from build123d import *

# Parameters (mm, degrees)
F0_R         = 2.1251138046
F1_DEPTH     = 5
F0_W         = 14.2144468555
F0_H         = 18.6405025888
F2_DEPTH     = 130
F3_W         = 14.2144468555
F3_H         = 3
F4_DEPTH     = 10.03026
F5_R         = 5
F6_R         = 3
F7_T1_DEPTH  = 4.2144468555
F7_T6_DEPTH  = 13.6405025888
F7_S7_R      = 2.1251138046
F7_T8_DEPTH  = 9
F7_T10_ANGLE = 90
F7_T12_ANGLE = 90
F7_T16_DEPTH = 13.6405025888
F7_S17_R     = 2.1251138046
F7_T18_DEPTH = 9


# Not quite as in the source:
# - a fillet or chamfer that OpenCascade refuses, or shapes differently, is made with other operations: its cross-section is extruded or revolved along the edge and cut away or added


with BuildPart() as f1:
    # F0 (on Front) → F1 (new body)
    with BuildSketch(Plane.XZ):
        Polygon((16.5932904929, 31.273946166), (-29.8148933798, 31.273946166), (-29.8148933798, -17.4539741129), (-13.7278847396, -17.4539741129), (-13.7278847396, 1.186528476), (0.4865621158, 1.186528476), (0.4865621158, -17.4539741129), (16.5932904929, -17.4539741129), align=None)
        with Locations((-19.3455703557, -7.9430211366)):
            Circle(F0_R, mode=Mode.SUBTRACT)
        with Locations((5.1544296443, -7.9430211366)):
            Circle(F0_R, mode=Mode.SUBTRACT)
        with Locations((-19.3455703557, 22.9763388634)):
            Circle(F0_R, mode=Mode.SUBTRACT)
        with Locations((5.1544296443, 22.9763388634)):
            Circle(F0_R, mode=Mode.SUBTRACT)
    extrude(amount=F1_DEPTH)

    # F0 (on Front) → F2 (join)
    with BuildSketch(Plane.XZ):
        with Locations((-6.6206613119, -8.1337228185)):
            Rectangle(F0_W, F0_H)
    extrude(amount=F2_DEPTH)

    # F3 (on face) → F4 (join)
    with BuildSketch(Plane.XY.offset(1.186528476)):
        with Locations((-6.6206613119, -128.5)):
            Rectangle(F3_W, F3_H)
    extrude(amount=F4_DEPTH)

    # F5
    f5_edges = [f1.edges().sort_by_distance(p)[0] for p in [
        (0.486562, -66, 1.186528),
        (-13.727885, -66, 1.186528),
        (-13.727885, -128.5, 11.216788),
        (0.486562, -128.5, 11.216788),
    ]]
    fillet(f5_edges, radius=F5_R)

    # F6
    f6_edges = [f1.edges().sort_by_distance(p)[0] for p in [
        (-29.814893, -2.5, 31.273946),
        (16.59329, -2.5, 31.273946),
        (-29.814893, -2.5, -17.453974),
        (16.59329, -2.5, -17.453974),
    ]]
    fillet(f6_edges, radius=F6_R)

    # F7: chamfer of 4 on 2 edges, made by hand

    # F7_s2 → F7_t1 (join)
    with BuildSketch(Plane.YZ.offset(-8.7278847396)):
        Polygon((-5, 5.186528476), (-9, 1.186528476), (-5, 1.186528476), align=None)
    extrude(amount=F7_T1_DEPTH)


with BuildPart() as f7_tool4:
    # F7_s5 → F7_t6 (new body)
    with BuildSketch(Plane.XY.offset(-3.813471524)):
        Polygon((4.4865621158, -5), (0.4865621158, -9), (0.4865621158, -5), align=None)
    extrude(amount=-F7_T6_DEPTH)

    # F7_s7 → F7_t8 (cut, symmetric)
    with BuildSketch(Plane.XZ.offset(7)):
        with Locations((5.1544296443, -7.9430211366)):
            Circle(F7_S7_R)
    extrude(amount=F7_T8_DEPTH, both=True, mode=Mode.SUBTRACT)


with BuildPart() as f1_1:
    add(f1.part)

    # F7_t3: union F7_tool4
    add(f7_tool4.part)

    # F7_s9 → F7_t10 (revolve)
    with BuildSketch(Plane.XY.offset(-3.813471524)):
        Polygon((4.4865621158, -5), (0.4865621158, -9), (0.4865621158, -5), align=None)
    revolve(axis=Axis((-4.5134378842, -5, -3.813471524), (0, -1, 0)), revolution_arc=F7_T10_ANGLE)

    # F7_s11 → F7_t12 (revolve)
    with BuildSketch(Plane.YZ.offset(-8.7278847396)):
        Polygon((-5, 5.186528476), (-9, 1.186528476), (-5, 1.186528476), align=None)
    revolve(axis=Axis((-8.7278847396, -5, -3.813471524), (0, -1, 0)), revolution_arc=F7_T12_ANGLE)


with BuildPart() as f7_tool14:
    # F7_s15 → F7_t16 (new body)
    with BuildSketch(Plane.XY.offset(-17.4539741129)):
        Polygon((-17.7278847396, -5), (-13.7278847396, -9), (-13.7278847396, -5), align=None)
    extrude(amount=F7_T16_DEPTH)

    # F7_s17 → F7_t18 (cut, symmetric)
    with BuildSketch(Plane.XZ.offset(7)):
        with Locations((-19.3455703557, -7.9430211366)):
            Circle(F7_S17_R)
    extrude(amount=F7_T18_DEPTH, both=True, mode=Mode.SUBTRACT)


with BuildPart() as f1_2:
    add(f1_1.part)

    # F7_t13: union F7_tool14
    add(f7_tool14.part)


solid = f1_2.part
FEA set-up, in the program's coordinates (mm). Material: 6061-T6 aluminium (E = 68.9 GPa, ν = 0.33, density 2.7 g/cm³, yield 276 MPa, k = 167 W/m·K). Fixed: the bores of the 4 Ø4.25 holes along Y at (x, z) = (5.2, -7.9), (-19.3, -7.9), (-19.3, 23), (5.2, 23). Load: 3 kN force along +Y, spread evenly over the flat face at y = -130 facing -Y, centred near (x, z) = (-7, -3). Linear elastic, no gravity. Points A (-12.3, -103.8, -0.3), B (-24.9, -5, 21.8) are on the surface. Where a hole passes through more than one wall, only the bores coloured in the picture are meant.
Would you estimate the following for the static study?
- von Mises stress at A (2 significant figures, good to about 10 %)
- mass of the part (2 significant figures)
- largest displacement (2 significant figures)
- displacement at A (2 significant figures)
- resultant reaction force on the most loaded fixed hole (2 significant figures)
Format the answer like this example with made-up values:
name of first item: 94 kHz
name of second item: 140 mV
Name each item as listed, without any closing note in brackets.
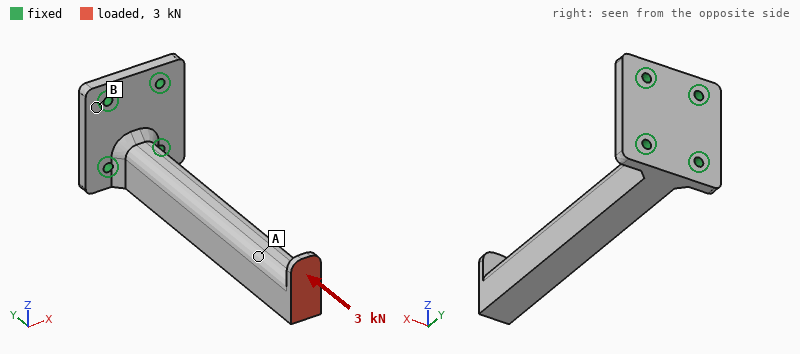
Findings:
von Mises stress at A: 30 MPa
mass of the part: 120 g
largest displacement: 0.39 mm
displacement at A: 0.21 mm
resultant reaction force on the most loaded fixed hole: 1.5 kN
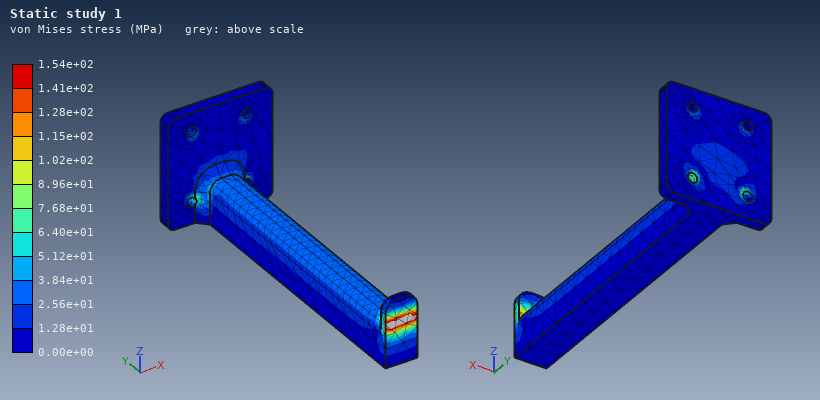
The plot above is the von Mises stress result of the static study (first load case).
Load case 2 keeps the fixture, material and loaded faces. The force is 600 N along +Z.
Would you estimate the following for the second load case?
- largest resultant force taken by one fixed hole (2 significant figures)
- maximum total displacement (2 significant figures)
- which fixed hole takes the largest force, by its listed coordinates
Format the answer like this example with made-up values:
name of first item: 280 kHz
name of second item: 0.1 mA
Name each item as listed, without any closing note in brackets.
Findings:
largest resultant force taken by one fixed hole: 1.1 kN
maximum total displacement: 1.3 mm
which fixed hole takes the largest force, by its listed coordinates: (5.2, -7.9)
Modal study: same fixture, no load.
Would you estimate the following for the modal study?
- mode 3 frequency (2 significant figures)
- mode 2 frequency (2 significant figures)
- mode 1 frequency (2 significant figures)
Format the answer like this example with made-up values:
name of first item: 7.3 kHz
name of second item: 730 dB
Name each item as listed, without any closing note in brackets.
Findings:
mode 3 frequency: 4000 Hz
mode 2 frequency: 680 Hz
mode 1 frequency: 670 Hz
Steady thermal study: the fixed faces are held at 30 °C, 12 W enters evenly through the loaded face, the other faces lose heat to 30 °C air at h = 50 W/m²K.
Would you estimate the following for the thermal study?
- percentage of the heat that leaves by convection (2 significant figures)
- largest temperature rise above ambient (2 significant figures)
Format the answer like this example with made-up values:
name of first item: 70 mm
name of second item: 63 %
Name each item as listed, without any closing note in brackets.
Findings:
percentage of the heat that leaves by convection: 43 %
largest temperature rise above ambient: 30 K
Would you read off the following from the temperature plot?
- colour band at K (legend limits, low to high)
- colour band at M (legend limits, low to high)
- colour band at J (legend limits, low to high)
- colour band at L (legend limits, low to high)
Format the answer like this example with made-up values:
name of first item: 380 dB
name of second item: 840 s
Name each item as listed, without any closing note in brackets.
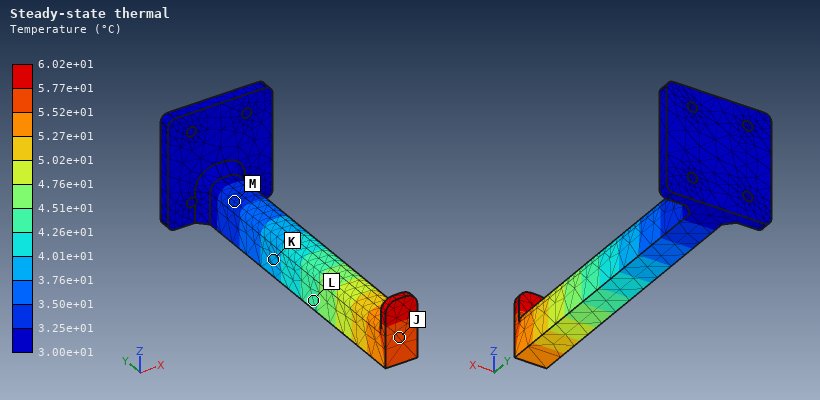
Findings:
colour band at K: 3.76e+01 to 4.01e+01 °C
colour band at M: 3.25e+01 to 3.50e+01 °C
colour band at J: 5.52e+01 to 5.77e+01 °C
colour band at L: 4.26e+01 to 4.51e+01 °C
